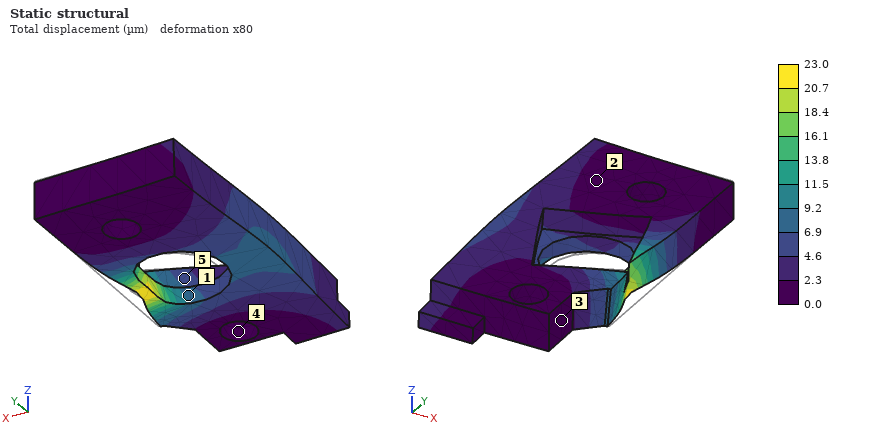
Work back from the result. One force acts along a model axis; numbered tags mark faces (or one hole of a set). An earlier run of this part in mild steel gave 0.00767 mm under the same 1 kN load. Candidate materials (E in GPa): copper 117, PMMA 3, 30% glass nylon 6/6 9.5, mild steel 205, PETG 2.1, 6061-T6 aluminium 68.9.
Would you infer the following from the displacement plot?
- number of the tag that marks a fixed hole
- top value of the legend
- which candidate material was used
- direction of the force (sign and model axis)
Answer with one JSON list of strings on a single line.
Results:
["4", "23.0 µm", "6061-T6 aluminium", "-X"]
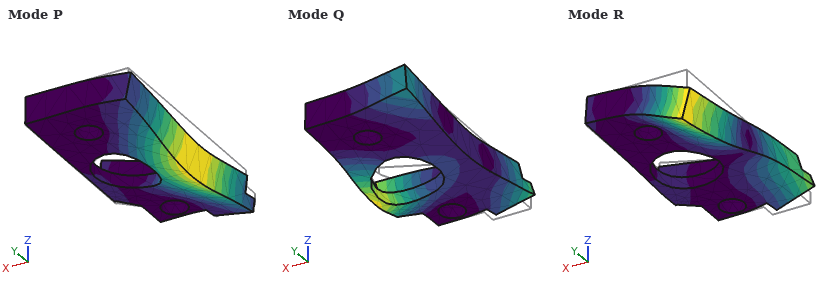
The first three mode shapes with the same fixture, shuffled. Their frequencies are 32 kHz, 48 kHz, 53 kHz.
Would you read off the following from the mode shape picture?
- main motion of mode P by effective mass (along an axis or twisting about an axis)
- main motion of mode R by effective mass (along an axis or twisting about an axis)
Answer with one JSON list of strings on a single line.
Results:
["along Z", "twisting about X"]
